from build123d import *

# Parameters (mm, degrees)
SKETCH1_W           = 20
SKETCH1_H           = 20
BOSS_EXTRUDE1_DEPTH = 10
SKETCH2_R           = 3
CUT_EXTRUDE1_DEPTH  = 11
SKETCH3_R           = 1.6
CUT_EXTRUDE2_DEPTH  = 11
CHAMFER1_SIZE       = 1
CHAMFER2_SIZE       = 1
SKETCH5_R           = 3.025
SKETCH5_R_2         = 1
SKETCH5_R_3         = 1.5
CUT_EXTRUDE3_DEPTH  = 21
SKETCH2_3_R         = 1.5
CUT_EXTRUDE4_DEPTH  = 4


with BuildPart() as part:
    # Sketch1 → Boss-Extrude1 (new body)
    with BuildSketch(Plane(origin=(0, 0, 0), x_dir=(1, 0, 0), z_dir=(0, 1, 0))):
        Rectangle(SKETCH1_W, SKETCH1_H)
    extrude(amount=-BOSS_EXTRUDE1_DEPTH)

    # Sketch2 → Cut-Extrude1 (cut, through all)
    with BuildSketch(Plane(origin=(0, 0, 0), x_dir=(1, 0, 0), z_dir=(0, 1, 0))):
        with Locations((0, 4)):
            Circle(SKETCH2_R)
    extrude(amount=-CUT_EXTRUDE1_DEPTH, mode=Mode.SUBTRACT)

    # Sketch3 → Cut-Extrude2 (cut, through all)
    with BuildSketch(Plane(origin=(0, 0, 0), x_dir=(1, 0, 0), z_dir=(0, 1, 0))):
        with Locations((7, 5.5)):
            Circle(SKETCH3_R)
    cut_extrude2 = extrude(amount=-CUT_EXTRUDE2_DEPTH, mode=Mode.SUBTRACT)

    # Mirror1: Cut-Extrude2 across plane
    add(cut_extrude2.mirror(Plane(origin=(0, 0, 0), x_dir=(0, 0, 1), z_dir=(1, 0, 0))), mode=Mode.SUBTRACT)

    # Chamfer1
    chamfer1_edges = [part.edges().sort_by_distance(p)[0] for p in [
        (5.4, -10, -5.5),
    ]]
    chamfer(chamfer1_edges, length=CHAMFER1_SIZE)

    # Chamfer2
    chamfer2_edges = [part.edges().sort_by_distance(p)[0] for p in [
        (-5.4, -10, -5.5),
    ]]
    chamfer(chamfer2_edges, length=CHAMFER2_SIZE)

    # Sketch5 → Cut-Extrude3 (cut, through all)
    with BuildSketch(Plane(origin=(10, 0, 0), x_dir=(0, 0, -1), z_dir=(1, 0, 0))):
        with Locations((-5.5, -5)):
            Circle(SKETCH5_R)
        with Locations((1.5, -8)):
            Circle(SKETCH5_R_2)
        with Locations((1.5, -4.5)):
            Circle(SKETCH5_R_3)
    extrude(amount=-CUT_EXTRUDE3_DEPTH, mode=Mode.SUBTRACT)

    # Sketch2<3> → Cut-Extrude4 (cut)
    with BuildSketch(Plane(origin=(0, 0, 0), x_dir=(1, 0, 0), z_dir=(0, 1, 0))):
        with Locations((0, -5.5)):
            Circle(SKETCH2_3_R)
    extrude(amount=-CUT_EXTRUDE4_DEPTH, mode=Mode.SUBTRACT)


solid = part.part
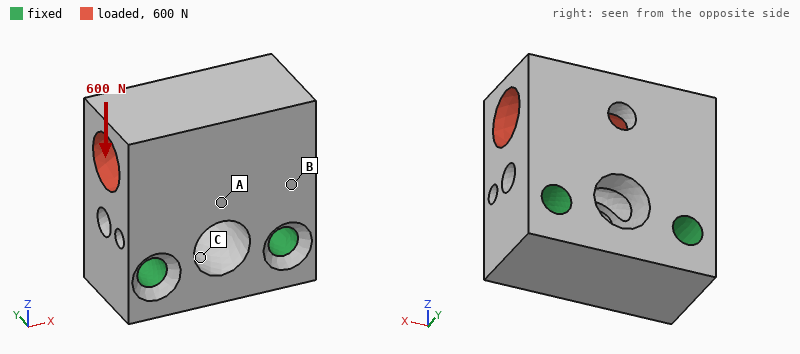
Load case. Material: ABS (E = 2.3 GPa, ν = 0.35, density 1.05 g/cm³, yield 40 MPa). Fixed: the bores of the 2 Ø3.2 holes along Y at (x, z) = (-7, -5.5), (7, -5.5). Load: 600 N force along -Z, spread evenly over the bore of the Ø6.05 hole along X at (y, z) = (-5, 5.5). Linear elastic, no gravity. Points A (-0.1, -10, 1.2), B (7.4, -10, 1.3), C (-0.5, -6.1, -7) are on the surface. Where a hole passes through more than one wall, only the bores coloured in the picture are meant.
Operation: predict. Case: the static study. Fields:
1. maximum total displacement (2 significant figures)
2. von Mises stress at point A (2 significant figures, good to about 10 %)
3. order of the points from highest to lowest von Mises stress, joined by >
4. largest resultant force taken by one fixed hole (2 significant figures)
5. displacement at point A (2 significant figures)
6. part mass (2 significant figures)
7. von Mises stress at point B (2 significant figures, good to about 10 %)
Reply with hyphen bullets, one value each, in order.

- 56 µm
- 3.2 MPa
- B > A > C
- 300 N
- 33 µm
- 2.9 g
- 7.7 MPa
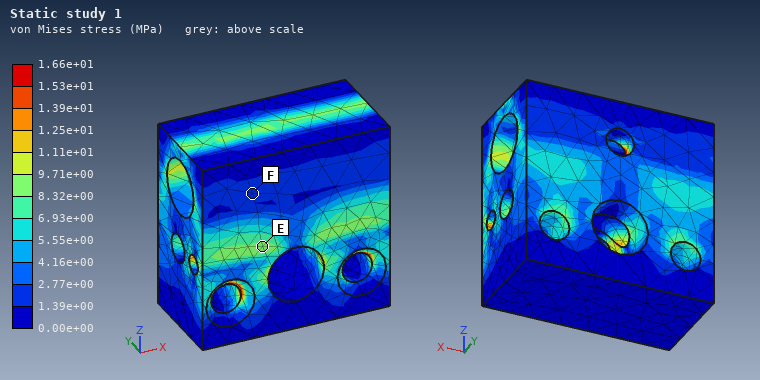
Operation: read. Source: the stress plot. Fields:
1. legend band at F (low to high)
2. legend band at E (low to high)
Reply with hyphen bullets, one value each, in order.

- 1.39e+00 to 2.77e+00 MPa
- 8.32e+00 to 9.71e+00 MPa
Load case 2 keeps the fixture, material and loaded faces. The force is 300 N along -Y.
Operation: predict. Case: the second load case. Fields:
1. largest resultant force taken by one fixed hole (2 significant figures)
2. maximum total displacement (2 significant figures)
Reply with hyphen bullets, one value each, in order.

- 150 N
- 0.20 mm
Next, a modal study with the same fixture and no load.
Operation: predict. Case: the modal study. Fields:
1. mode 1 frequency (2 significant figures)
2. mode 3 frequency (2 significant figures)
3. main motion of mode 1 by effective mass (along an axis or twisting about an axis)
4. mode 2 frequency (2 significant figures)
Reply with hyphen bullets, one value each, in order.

- 6200 Hz
- 10 kHz
- along Y
- 9900 Hz
